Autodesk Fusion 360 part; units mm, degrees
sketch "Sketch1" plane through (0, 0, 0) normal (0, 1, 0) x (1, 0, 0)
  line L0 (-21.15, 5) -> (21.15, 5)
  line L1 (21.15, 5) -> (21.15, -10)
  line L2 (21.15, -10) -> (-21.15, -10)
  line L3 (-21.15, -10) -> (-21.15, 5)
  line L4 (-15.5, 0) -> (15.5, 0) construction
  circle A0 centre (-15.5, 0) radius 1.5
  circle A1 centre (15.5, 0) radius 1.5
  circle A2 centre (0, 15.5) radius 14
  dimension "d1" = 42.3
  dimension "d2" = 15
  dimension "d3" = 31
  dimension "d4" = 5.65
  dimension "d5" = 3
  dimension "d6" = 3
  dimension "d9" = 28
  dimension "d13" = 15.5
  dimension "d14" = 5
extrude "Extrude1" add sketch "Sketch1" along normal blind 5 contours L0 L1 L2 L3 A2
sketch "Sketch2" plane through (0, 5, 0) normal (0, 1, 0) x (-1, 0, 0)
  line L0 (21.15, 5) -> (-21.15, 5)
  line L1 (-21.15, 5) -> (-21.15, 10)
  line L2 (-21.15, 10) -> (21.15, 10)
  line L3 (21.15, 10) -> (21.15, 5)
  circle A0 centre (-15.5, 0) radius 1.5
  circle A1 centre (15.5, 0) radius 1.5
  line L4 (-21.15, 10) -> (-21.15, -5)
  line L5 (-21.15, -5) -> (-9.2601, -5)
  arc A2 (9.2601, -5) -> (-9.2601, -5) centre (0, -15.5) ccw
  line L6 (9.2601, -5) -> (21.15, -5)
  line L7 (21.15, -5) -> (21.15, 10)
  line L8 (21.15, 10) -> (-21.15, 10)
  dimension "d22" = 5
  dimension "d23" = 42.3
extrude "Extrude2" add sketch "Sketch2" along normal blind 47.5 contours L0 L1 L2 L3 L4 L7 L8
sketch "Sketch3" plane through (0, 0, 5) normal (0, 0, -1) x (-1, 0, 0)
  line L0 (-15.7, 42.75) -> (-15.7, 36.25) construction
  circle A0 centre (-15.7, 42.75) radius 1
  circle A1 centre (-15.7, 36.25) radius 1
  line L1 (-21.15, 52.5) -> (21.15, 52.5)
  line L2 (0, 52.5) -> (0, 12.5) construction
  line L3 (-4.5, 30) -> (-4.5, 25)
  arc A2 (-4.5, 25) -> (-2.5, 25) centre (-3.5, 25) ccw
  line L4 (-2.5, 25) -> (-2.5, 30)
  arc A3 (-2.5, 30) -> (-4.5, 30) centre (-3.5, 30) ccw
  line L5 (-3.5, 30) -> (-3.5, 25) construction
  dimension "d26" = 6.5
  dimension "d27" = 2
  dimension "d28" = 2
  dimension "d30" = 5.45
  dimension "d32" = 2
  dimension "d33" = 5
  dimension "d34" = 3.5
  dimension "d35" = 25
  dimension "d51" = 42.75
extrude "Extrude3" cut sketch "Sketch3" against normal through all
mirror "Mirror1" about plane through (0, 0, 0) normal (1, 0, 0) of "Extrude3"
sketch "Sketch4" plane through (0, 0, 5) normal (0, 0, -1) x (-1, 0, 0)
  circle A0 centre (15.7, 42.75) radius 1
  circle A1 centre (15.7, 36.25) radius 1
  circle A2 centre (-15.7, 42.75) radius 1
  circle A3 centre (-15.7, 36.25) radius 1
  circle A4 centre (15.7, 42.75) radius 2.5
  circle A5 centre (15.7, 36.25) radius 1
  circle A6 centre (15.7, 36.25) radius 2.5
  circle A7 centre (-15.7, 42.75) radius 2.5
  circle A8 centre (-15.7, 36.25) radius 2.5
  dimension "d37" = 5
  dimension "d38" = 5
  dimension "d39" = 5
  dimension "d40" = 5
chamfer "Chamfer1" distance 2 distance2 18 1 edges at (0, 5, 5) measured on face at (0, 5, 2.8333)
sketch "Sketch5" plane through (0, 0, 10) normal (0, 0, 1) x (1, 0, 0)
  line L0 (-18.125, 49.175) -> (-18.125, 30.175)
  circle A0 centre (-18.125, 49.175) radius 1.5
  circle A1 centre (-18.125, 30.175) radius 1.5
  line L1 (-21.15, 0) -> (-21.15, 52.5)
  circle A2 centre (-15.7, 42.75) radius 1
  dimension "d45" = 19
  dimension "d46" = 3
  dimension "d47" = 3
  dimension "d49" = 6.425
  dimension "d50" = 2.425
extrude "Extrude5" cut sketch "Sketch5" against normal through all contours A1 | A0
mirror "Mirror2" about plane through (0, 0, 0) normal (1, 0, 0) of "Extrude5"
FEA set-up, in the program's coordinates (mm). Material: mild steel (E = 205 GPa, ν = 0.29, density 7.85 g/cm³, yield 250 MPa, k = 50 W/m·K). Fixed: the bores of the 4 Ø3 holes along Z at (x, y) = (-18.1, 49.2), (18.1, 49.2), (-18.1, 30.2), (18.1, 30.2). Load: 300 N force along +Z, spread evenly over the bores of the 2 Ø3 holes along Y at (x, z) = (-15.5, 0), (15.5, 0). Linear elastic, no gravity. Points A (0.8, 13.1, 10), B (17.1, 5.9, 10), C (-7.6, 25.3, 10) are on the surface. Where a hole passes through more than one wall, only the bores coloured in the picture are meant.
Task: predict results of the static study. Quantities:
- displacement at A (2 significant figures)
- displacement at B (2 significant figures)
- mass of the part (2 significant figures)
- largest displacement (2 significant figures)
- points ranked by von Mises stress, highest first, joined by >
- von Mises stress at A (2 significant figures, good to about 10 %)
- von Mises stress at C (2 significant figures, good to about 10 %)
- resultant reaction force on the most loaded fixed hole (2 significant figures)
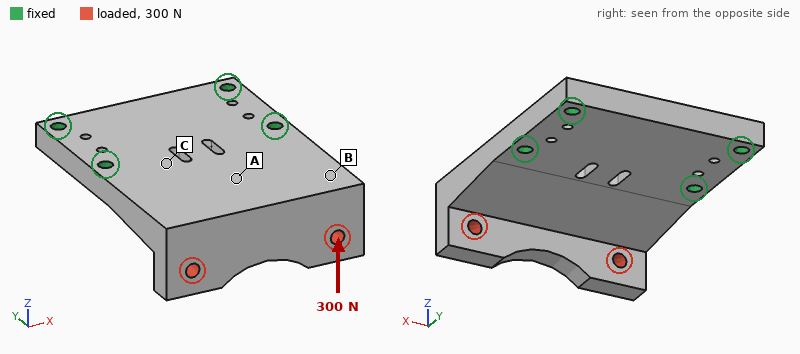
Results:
15 µm
23 µm
100 g
35 µm
C > A > B
12 MPa
32 MPa
230 N
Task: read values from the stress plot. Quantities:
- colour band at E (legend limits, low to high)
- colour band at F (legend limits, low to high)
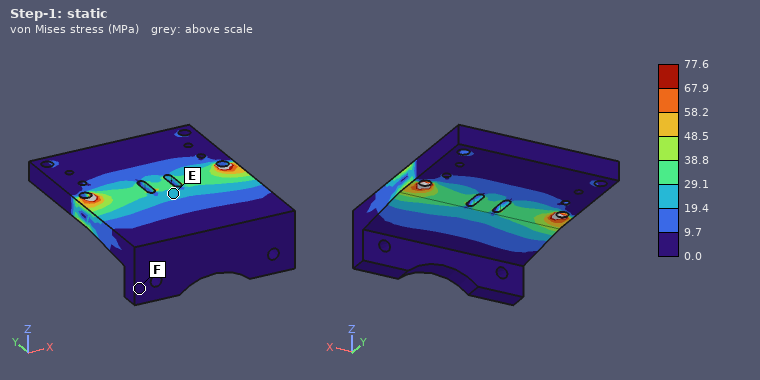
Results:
19.4 to 29.1 MPa
0.0 to 9.7 MPa
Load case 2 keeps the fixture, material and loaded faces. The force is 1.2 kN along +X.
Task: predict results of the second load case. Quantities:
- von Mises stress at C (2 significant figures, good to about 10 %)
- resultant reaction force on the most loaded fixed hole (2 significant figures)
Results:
7.6 MPa
1.1 kN
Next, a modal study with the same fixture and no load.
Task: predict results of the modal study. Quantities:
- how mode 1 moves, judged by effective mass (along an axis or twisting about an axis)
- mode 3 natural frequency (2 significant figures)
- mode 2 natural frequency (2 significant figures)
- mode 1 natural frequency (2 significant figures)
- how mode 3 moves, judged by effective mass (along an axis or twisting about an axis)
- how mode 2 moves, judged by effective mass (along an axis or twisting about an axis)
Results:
along Z
14 kHz
6900 Hz
2800 Hz
along X
twisting about Y
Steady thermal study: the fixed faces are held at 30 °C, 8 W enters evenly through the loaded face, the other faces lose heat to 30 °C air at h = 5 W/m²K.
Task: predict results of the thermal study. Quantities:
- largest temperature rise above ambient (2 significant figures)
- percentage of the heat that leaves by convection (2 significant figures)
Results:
29 K
4.2 %
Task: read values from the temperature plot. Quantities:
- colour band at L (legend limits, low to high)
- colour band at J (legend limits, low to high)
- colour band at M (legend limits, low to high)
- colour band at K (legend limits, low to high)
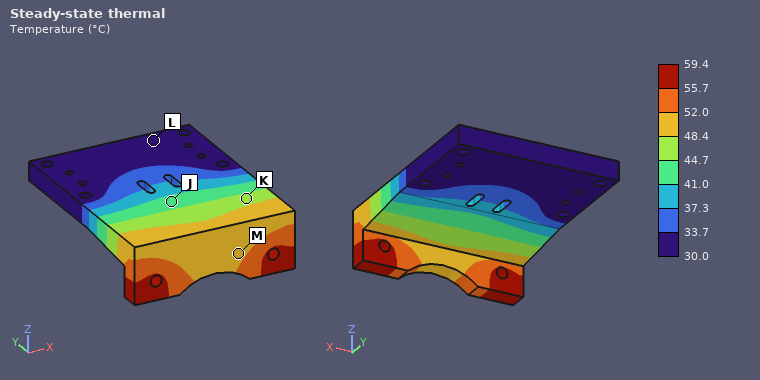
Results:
30.0 to 33.7 °C
41.0 to 44.7 °C
48.4 to 52.0 °C
44.7 to 48.4 °C
